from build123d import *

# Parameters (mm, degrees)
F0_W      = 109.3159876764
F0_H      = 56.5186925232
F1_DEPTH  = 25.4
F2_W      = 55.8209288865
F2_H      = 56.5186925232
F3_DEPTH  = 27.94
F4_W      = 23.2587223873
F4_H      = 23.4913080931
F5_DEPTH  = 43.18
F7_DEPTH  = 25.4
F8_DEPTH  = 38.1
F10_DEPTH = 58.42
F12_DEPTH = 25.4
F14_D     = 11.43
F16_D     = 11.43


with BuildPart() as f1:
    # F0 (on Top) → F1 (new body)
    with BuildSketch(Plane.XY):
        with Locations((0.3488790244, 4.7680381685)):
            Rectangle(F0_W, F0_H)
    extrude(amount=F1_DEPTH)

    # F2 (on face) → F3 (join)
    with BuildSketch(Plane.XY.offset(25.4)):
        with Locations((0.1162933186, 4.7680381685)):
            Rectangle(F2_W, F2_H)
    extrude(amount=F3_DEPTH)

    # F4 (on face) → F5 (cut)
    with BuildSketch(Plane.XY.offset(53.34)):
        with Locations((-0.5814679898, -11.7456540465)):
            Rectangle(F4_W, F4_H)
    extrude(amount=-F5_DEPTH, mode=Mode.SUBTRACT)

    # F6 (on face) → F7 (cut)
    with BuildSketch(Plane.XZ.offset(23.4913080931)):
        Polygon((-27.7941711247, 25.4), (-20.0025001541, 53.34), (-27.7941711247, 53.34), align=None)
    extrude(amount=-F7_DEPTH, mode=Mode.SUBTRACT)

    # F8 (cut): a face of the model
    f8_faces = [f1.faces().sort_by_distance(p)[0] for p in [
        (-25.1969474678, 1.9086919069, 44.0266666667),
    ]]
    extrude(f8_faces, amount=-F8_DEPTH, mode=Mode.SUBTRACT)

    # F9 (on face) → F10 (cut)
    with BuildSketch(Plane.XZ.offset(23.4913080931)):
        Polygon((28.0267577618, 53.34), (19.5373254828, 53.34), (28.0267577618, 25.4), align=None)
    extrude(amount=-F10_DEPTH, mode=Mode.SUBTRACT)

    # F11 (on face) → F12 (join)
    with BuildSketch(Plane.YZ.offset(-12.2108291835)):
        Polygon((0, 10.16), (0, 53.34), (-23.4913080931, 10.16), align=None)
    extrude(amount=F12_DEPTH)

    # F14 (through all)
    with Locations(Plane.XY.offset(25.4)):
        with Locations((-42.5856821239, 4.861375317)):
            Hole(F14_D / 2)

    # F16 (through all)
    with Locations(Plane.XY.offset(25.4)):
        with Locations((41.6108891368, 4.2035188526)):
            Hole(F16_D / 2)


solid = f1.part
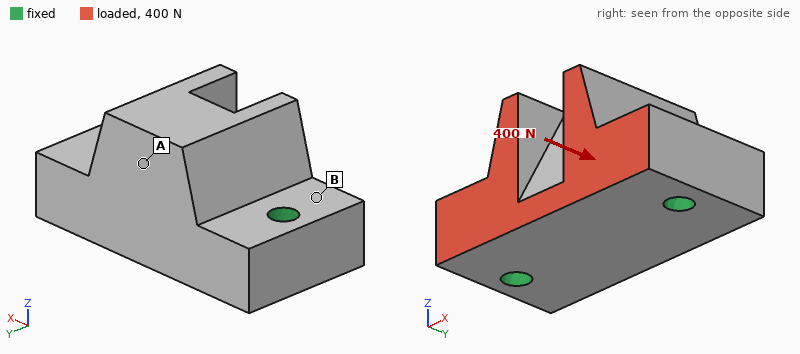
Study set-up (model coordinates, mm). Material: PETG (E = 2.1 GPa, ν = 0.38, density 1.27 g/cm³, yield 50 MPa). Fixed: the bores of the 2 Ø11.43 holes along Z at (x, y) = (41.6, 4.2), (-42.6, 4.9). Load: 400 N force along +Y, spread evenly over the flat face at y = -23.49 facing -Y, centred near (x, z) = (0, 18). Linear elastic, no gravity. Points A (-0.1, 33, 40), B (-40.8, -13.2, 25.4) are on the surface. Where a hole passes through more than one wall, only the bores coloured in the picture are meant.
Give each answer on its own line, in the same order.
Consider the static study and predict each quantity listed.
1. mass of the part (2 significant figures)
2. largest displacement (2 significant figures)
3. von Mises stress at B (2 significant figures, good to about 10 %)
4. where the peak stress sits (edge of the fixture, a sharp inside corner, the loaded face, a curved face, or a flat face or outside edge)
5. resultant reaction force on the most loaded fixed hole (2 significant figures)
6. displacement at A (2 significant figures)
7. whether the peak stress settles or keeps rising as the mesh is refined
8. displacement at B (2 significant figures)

270 g
14 µm
0.23 MPa
edge of the fixture
210 N
9.7 µm
keeps rising
2.7 µm
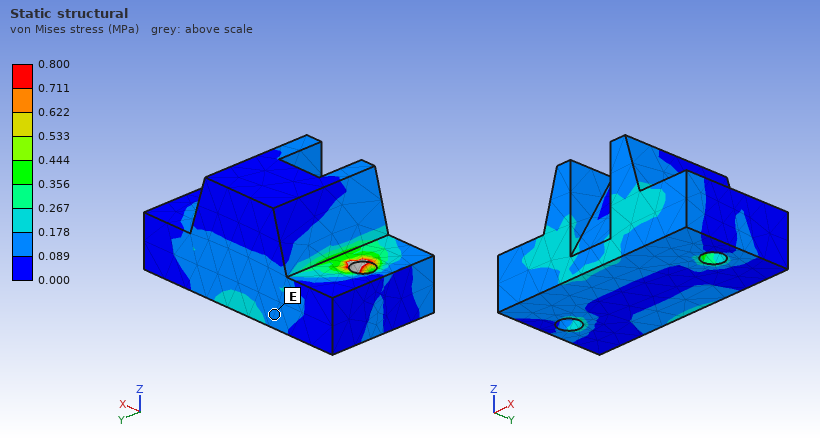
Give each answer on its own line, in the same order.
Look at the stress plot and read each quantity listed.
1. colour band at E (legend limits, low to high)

0.089 to 0.178 MPa
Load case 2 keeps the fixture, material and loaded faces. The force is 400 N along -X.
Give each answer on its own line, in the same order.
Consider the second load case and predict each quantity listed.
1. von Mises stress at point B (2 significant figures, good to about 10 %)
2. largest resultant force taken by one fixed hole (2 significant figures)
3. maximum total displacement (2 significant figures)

0.27 MPa
240 N
21 µm
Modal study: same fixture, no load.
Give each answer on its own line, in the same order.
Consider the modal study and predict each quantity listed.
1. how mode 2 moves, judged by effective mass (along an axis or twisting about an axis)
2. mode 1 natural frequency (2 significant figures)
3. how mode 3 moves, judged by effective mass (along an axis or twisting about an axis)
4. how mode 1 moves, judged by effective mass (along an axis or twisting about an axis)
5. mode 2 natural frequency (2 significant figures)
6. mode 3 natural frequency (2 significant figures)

along Z
1600 Hz
along Y
along Y
2500 Hz
3100 Hz
